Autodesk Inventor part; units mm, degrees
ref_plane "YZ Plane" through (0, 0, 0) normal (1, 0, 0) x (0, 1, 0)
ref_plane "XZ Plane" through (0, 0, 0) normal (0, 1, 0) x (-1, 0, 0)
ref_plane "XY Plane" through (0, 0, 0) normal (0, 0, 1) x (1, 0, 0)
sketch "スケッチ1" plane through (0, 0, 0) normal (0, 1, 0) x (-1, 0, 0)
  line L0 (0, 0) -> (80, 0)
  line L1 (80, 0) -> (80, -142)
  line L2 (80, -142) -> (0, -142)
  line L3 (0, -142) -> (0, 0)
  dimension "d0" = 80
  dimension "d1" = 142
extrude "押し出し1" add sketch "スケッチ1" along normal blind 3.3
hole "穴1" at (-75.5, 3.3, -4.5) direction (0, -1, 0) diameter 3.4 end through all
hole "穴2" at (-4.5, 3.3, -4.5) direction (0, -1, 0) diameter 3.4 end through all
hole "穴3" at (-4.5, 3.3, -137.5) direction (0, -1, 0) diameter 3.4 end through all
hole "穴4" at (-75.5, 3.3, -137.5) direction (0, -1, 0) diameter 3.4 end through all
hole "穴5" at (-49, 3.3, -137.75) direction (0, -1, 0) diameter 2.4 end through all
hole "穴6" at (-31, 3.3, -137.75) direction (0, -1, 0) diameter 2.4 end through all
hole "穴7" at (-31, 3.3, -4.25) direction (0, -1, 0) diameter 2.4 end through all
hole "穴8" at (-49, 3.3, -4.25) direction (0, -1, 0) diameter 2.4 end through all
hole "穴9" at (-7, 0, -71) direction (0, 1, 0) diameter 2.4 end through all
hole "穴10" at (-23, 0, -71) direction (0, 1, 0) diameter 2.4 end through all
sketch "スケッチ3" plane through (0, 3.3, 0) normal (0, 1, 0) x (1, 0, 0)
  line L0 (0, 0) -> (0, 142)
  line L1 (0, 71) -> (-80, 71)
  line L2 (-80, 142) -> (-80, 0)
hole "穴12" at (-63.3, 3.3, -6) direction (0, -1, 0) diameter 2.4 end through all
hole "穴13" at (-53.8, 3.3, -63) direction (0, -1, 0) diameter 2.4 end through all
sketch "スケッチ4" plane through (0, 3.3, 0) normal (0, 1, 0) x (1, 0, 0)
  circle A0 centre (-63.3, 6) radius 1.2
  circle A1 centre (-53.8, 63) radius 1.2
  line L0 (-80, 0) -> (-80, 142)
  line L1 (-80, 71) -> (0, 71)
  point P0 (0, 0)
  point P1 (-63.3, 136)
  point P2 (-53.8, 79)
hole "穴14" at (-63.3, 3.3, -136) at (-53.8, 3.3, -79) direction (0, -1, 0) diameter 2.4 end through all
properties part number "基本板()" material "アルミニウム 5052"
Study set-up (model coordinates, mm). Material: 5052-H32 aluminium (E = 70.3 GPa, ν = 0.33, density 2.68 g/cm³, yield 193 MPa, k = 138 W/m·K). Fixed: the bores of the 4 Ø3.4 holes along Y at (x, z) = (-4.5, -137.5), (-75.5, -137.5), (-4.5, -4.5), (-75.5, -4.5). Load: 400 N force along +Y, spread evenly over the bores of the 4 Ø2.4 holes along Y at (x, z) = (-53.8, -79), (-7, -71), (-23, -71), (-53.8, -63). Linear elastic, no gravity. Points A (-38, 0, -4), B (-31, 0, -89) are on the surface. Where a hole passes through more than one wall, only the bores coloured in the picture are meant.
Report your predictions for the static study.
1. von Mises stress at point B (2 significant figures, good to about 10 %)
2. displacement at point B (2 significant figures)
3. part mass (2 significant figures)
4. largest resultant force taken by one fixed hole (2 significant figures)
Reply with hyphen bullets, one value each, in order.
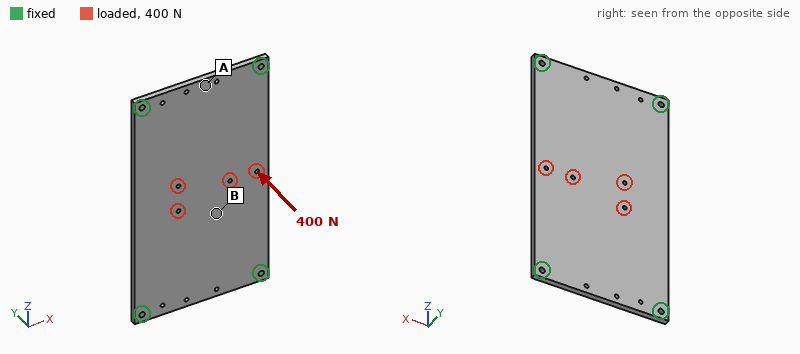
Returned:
- 26 MPa
- 0.36 mm
- 100 g
- 120 N
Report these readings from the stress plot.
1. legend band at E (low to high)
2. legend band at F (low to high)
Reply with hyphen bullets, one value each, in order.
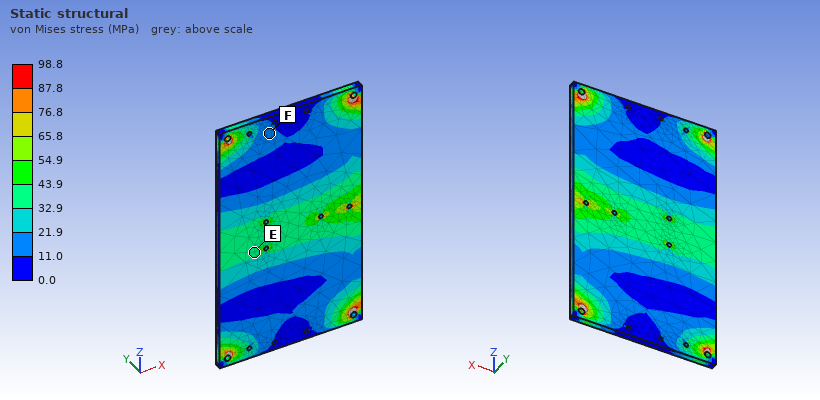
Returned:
- 32.9 to 43.9 MPa
- 11.0 to 21.9 MPa
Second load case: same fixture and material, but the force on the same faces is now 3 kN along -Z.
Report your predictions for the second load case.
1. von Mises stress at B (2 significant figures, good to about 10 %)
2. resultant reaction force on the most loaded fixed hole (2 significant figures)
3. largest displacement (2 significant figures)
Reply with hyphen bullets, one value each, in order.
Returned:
- 4.1 MPa
- 810 N
- 11 µm
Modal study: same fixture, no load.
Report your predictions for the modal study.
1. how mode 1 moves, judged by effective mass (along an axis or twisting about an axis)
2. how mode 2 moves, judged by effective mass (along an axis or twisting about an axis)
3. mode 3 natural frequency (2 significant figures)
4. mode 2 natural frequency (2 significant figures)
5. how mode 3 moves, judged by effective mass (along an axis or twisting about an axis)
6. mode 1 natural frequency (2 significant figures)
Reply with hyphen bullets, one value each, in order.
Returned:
- along Y
- twisting about Z
- 2200 Hz
- 1400 Hz
- twisting about X
- 790 Hz
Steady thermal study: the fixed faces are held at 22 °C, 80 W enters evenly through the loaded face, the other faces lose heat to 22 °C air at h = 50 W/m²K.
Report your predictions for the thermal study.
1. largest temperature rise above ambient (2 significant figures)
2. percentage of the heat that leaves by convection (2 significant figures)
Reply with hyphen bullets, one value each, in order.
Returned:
- 76 K
- 49 %
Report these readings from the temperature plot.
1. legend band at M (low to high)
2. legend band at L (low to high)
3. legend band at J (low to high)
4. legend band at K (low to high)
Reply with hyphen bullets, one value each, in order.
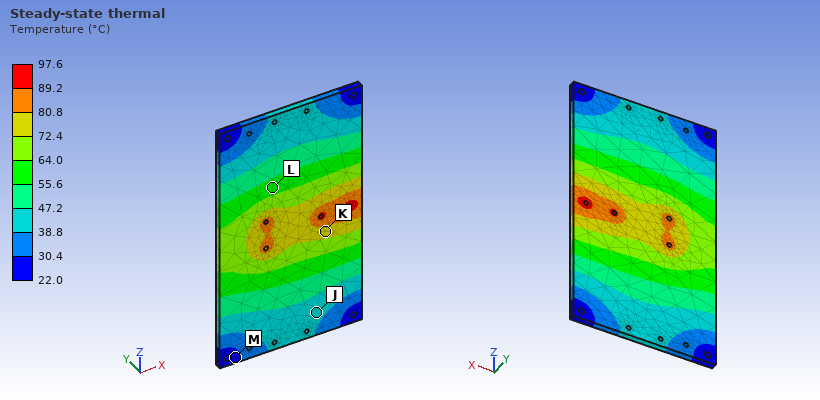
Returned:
- 22.0 to 30.4 °C
- 55.6 to 64.0 °C
- 38.8 to 47.2 °C
- 72.4 to 80.8 °C
